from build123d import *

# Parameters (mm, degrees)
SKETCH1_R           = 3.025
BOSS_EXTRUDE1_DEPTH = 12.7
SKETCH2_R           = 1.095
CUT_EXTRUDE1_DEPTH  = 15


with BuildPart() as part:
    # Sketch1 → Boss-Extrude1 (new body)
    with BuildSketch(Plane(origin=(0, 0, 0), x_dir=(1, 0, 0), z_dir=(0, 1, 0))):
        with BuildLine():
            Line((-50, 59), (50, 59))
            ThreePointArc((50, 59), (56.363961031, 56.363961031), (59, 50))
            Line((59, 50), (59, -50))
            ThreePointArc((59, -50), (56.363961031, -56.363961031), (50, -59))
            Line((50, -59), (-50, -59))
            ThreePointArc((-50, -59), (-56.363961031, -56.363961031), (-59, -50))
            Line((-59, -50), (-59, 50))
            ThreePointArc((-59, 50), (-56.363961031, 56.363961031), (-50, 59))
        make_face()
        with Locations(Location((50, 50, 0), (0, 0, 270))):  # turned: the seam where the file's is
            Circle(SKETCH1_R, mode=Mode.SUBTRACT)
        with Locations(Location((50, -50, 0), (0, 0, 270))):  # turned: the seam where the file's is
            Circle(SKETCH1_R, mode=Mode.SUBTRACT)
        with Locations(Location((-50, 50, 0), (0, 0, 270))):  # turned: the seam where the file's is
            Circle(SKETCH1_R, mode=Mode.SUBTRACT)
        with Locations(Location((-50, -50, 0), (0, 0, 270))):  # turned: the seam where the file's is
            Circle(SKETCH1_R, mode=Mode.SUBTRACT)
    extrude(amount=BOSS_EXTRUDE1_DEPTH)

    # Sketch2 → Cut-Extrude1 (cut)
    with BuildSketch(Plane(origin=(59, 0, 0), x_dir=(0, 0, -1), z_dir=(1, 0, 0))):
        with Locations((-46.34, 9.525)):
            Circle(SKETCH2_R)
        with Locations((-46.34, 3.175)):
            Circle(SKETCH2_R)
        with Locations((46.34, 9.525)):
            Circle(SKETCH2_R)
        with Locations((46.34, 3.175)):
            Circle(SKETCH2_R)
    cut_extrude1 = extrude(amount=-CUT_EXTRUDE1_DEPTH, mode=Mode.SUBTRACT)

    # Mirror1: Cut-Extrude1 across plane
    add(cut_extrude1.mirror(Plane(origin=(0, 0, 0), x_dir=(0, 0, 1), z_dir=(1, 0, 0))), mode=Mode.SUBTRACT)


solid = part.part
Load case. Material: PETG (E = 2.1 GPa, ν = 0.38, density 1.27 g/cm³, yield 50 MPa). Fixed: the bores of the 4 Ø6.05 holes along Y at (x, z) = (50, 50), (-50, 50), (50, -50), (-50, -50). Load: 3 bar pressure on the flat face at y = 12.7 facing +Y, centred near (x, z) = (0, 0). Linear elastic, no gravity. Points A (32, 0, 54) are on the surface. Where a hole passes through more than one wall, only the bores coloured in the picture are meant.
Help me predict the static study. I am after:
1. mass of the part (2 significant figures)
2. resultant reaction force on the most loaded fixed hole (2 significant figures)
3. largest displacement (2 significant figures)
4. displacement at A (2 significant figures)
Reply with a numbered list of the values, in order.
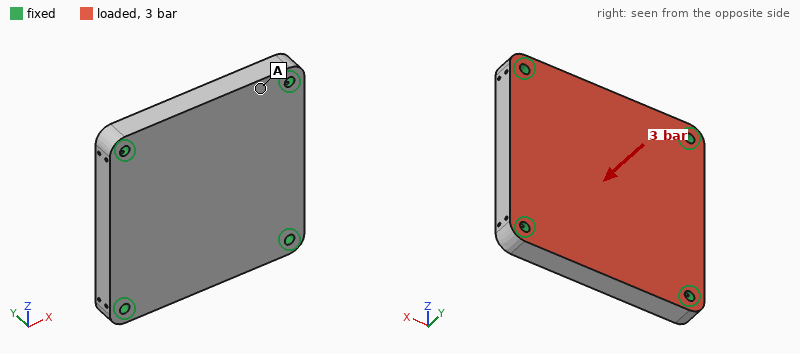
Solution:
1. 220 g
2. 1.0 kN
3. 0.73 mm
4. 0.18 mm
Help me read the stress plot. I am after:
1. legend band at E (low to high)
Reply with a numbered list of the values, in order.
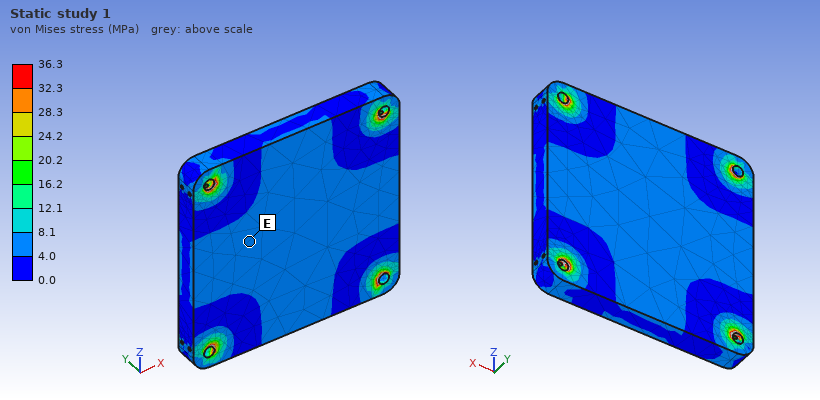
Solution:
1. 4.0 to 8.1 MPa
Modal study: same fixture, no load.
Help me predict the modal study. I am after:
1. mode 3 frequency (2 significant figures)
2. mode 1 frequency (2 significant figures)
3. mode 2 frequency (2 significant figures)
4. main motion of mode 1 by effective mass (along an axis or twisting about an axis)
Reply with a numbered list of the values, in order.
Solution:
1. 1600 Hz
2. 950 Hz
3. 1600 Hz
4. along Y
